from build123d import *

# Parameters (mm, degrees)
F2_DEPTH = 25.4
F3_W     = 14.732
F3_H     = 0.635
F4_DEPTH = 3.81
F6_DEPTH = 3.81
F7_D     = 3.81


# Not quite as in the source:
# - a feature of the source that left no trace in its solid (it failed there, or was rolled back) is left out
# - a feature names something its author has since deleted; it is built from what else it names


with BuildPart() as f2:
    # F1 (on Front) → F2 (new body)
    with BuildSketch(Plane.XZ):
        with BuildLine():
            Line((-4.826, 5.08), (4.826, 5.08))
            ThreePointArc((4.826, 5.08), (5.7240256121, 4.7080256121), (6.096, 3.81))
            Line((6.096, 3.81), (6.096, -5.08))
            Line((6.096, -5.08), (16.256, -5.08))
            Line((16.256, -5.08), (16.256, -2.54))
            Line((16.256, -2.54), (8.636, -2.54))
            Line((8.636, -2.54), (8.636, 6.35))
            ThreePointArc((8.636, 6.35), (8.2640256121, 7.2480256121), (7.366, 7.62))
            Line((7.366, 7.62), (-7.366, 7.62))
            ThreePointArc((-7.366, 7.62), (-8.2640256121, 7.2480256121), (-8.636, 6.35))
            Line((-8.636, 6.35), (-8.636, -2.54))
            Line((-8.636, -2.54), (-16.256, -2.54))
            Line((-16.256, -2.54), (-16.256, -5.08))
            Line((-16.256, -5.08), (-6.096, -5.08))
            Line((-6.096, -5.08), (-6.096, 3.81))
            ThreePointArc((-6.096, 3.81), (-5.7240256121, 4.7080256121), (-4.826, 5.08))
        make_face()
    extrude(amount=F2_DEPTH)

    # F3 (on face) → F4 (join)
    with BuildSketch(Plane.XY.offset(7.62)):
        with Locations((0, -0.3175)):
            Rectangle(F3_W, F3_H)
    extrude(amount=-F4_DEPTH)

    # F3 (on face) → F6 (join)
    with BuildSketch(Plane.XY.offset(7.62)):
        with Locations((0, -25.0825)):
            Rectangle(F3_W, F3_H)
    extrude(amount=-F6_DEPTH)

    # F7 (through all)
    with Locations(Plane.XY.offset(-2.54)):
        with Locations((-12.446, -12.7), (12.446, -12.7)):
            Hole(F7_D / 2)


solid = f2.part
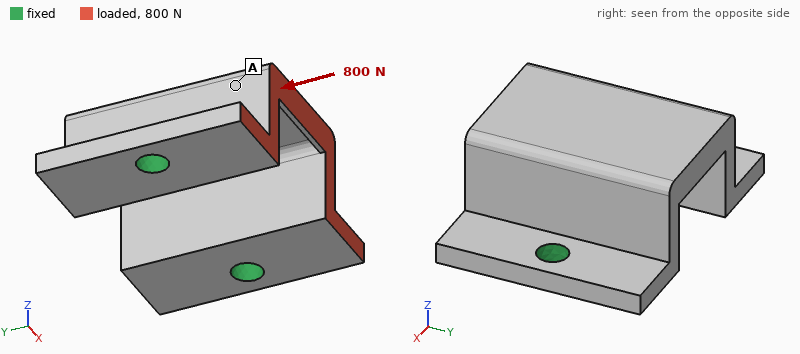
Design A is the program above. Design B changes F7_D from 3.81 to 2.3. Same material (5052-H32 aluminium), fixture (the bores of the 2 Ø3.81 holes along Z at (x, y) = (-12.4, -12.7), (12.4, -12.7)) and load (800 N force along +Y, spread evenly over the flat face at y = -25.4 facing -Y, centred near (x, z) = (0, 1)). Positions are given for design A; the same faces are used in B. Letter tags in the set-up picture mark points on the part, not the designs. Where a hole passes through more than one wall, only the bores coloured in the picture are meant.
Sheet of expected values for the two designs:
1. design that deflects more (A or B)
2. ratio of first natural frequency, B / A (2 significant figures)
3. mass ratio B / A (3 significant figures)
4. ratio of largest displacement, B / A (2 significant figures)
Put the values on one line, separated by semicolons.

B; 0.77; 1.01; 1.7
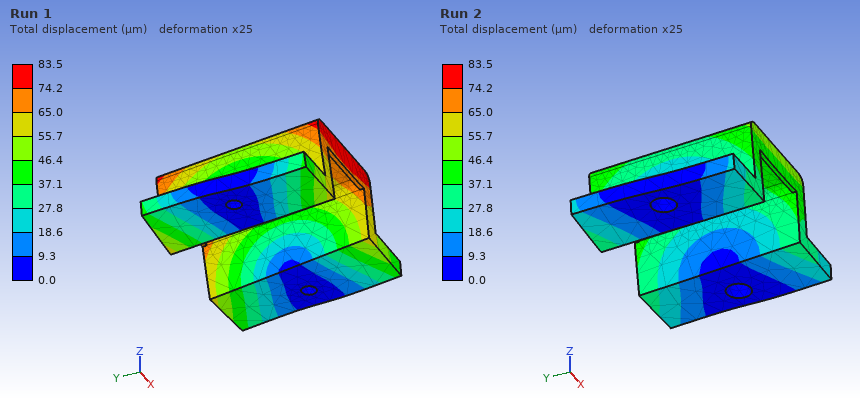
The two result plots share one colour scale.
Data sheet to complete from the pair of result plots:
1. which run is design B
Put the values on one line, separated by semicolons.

Run 1
